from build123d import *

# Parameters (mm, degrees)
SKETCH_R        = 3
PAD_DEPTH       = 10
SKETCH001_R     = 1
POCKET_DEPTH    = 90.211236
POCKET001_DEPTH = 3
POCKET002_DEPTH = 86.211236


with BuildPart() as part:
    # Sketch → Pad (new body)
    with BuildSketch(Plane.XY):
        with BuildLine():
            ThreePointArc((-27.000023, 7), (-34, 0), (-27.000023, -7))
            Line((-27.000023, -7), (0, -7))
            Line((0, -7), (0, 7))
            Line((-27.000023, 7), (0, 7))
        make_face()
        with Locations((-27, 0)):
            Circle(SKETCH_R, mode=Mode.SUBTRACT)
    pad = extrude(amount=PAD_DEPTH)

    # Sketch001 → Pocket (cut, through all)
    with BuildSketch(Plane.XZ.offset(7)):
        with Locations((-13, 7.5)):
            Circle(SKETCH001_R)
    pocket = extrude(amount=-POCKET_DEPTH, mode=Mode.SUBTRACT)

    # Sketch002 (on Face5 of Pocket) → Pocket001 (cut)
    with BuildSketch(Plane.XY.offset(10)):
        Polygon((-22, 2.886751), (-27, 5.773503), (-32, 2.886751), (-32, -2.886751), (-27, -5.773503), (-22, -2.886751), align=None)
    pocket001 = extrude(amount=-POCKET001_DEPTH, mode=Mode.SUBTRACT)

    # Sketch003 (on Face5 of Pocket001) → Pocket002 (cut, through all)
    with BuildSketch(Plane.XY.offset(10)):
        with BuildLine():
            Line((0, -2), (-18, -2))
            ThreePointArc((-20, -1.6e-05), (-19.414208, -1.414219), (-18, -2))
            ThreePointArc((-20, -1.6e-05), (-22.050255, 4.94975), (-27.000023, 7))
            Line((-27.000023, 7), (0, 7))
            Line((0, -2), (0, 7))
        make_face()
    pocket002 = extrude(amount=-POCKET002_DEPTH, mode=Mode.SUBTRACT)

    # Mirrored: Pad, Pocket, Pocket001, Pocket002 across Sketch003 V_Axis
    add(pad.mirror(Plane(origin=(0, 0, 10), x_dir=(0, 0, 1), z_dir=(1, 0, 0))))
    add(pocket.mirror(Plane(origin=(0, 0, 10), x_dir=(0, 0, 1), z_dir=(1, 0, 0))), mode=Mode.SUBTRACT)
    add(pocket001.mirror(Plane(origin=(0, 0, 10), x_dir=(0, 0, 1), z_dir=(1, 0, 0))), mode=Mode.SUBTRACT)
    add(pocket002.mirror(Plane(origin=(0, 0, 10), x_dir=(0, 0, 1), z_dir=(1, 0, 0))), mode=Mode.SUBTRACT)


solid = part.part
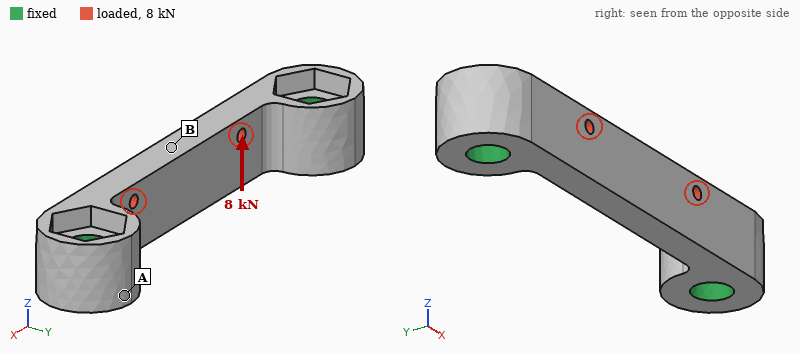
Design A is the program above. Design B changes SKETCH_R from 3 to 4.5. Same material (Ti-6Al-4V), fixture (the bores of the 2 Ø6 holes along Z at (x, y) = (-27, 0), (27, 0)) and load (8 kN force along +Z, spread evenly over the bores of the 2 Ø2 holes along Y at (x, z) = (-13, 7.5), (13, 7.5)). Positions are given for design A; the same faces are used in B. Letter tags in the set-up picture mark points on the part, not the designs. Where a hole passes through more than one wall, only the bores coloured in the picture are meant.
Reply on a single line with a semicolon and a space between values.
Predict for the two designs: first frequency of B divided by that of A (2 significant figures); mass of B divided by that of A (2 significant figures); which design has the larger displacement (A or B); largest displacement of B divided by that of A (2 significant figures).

1.1; 0.89; A; 0.77
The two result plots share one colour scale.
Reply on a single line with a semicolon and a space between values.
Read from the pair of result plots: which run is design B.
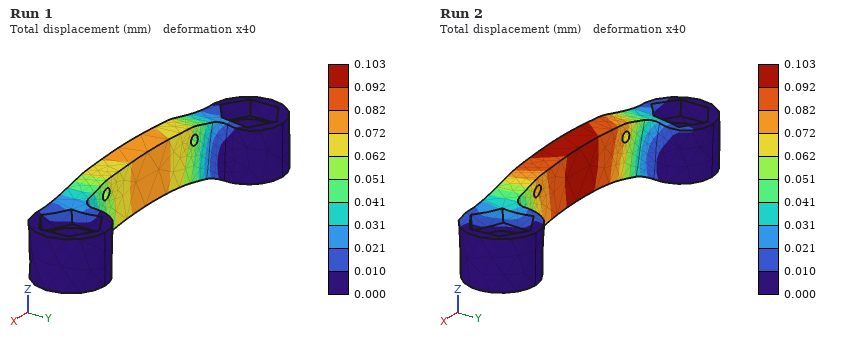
Run 1
